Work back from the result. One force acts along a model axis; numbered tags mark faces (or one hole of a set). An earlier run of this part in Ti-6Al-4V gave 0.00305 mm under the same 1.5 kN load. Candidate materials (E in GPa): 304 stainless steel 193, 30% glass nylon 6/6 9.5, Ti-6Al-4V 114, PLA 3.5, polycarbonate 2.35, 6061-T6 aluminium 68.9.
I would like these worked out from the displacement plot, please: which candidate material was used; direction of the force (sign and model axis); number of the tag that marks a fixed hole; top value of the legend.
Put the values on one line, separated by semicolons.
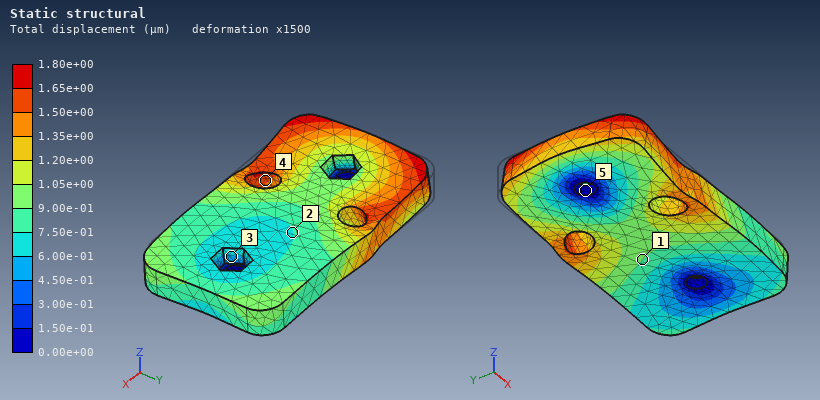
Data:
304 stainless steel; +X; 5; 1.80e+00 µm
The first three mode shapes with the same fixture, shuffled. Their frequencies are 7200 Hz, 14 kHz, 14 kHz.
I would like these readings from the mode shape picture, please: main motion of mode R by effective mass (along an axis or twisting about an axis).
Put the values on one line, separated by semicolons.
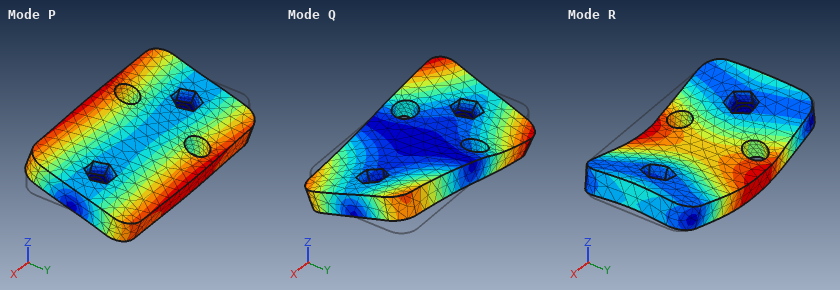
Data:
along Z
